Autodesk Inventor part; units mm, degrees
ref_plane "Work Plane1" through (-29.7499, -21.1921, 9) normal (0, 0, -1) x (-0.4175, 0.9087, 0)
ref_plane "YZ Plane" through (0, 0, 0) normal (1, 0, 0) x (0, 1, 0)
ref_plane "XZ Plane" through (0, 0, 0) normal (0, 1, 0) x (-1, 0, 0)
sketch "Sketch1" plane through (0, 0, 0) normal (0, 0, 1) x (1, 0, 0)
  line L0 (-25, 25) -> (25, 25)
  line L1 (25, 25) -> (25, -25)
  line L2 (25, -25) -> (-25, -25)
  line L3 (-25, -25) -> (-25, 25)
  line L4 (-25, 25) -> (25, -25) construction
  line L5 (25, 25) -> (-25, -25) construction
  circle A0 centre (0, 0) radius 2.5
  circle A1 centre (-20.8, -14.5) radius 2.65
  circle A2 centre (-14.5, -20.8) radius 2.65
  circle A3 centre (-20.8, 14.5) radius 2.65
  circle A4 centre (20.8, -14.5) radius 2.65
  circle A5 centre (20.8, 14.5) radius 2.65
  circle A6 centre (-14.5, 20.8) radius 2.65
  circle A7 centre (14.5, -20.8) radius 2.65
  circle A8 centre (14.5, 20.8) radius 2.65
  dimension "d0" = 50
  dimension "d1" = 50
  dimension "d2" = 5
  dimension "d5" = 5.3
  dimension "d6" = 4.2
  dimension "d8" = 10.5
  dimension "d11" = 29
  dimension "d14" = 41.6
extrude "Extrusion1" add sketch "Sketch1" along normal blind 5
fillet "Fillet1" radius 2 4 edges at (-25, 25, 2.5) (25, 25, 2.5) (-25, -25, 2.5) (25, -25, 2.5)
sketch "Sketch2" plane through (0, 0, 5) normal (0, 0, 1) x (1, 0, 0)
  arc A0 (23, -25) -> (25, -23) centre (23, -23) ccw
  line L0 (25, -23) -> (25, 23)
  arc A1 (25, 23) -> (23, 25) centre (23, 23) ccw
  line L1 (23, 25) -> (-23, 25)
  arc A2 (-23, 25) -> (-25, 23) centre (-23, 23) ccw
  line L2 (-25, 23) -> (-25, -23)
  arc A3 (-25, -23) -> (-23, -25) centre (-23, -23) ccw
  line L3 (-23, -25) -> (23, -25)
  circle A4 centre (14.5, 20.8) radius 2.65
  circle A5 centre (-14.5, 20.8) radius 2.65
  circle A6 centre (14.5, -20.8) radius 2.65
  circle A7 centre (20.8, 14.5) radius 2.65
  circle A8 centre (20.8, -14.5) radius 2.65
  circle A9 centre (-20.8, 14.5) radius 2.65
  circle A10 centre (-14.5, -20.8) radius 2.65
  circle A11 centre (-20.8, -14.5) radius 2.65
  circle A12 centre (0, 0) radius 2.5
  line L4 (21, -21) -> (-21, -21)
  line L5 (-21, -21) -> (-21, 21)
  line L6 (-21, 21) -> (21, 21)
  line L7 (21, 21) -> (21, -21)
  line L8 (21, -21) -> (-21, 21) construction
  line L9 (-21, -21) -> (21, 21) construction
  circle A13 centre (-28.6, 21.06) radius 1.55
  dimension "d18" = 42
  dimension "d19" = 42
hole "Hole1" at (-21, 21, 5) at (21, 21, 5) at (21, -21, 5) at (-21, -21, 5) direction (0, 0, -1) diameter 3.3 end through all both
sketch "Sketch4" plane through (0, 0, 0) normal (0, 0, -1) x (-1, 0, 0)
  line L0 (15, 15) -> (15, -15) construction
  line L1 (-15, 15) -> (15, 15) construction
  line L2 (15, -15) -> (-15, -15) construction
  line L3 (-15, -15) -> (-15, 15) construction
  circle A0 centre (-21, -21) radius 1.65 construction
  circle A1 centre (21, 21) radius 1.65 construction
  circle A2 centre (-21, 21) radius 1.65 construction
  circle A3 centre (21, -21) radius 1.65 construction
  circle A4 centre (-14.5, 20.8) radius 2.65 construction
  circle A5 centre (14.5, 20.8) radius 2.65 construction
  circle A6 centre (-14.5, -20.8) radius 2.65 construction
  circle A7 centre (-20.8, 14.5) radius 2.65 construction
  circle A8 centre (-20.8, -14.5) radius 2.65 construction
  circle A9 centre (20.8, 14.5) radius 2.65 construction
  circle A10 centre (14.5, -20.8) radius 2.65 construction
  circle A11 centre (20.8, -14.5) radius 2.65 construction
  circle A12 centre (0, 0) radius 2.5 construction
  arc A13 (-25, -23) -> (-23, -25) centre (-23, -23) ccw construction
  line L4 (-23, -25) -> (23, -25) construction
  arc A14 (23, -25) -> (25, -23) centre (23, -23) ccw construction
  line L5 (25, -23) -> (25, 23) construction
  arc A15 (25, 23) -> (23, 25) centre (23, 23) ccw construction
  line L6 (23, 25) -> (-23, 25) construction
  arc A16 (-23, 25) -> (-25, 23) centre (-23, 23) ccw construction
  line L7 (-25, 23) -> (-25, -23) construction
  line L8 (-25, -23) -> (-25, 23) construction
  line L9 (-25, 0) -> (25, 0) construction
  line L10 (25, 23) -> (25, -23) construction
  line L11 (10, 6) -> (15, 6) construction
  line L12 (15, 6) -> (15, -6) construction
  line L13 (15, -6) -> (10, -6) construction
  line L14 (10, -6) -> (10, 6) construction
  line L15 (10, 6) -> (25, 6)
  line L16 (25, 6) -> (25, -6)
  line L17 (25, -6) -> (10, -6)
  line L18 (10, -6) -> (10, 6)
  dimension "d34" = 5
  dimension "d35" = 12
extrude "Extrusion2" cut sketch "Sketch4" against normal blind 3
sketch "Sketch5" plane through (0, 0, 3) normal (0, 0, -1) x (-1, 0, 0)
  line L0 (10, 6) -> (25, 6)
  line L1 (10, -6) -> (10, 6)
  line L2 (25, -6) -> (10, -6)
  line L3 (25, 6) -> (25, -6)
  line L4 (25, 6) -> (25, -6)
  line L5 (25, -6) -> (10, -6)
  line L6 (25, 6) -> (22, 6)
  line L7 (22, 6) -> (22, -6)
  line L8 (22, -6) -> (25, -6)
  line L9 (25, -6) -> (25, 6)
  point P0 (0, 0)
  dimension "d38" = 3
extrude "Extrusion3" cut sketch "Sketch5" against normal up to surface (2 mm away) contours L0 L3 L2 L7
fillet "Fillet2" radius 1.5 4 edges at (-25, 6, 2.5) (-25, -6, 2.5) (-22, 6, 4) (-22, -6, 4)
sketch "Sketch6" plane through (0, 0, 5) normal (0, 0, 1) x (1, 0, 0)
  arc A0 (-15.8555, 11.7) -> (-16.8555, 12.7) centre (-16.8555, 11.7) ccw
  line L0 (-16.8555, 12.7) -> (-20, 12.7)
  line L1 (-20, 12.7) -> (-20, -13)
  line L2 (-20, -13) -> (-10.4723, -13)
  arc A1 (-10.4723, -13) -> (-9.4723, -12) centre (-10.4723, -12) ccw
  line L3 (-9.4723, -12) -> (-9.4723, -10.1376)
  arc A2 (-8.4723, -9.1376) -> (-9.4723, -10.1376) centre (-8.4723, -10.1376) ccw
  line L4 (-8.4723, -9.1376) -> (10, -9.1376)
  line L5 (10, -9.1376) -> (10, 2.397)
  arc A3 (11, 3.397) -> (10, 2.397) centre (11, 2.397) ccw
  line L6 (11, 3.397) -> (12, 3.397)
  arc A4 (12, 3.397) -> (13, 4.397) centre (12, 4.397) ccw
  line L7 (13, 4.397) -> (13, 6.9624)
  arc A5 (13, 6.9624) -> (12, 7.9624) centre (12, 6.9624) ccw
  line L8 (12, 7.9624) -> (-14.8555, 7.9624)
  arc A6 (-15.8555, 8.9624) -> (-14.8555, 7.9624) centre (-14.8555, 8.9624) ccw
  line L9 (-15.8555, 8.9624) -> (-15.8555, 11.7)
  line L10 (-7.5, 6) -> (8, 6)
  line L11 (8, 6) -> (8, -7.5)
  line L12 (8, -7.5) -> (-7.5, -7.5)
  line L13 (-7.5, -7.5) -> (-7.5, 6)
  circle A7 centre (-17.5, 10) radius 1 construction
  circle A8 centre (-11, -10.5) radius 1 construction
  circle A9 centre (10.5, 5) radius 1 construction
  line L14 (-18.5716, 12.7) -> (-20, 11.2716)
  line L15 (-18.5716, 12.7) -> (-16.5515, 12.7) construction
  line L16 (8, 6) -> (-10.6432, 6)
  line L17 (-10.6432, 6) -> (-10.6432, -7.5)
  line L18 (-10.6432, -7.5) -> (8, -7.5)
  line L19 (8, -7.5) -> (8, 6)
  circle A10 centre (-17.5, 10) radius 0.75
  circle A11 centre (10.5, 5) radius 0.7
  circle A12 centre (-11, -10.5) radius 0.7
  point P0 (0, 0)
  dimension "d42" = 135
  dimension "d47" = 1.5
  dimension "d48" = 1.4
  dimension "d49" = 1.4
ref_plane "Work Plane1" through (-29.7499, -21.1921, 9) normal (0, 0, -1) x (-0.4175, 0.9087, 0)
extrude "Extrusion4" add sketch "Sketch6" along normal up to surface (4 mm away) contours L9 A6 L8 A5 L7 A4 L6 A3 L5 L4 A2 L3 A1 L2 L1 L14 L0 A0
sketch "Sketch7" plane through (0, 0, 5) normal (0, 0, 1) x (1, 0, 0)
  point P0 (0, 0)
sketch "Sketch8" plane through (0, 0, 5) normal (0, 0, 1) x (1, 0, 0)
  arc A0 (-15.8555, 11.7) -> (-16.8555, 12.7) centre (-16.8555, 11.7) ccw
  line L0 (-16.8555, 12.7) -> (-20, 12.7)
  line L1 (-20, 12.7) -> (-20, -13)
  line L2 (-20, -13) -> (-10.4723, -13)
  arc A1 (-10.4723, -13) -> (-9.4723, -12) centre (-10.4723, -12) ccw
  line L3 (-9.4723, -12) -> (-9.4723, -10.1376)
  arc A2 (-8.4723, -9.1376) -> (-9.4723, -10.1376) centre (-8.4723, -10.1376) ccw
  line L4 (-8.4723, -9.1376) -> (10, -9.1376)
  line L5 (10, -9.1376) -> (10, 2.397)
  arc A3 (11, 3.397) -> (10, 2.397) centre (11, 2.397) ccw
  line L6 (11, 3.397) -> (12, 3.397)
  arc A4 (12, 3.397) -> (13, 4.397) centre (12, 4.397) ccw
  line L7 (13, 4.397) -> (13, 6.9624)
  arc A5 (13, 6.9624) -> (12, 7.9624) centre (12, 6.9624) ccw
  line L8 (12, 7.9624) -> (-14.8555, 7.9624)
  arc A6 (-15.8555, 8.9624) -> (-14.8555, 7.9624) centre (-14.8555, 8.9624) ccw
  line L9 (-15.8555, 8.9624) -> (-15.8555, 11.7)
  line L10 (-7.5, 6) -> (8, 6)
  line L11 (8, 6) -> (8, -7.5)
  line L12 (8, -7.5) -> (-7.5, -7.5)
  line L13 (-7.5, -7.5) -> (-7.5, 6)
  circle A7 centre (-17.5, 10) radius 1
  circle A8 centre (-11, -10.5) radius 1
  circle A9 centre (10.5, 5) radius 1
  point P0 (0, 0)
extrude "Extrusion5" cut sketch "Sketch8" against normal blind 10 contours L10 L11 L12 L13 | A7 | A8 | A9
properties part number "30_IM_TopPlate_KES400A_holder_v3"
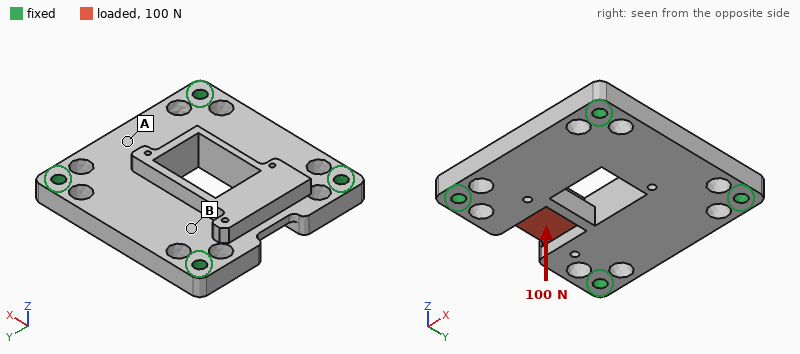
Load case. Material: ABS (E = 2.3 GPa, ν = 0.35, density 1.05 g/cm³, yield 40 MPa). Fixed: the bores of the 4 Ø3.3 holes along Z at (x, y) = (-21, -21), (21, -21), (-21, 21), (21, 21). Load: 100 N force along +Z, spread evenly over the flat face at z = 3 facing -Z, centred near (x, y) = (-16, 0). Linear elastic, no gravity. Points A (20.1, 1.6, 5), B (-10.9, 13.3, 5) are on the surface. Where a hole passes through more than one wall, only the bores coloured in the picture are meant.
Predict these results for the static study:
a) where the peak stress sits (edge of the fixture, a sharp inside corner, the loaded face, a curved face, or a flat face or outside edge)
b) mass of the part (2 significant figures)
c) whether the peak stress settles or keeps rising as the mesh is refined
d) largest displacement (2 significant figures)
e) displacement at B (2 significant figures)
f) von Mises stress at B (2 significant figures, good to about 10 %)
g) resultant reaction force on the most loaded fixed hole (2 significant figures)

edge of the fixture
12 g
keeps rising
0.11 mm
0.048 mm
1.6 MPa
64 N
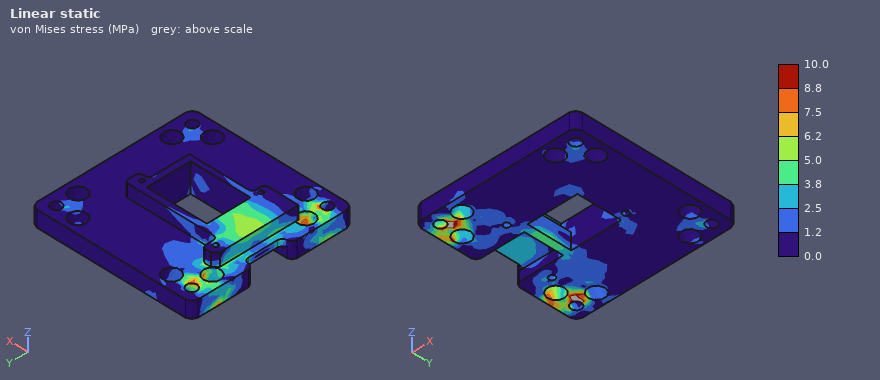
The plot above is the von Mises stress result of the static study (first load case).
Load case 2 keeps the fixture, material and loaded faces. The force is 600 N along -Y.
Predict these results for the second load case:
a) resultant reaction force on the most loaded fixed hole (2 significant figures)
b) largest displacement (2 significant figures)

250 N
91 µm
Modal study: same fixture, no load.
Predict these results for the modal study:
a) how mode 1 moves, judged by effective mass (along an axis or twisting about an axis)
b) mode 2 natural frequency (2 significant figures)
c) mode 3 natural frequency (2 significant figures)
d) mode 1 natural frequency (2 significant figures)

along Z
3900 Hz
4000 Hz
2600 Hz
